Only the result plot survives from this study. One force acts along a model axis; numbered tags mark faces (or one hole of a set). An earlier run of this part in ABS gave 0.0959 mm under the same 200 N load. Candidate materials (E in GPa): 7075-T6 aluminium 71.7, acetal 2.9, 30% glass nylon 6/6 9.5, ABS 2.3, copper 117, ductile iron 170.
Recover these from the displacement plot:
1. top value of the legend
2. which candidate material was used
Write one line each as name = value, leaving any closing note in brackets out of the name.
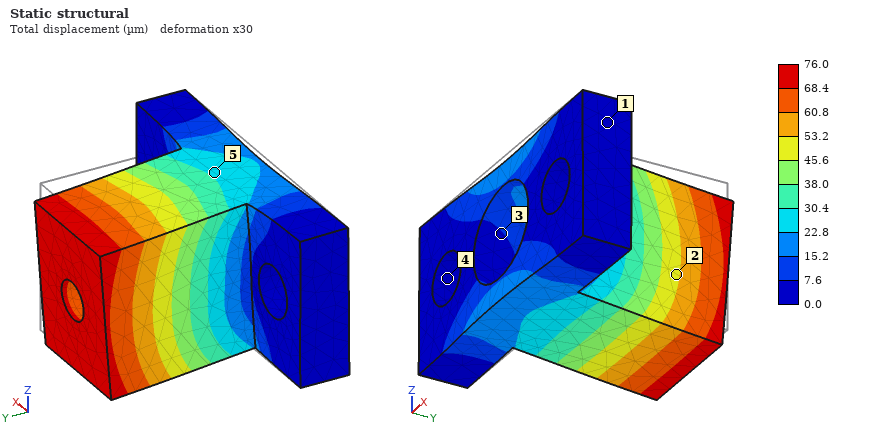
top value of the legend = 76.0 µm
which candidate material was used = acetal
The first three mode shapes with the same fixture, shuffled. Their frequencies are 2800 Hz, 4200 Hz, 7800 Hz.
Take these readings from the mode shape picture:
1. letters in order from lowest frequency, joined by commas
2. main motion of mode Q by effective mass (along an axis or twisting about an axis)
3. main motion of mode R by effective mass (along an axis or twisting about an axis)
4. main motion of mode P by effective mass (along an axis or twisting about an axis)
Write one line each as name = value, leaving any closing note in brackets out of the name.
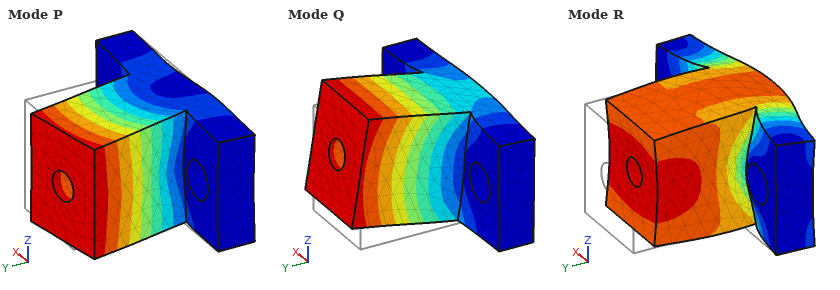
letters in order from lowest frequency, joined by commas = Q, P, R
main motion of mode Q by effective mass = along Z
main motion of mode R by effective mass = along Y
main motion of mode P by effective mass = along X
